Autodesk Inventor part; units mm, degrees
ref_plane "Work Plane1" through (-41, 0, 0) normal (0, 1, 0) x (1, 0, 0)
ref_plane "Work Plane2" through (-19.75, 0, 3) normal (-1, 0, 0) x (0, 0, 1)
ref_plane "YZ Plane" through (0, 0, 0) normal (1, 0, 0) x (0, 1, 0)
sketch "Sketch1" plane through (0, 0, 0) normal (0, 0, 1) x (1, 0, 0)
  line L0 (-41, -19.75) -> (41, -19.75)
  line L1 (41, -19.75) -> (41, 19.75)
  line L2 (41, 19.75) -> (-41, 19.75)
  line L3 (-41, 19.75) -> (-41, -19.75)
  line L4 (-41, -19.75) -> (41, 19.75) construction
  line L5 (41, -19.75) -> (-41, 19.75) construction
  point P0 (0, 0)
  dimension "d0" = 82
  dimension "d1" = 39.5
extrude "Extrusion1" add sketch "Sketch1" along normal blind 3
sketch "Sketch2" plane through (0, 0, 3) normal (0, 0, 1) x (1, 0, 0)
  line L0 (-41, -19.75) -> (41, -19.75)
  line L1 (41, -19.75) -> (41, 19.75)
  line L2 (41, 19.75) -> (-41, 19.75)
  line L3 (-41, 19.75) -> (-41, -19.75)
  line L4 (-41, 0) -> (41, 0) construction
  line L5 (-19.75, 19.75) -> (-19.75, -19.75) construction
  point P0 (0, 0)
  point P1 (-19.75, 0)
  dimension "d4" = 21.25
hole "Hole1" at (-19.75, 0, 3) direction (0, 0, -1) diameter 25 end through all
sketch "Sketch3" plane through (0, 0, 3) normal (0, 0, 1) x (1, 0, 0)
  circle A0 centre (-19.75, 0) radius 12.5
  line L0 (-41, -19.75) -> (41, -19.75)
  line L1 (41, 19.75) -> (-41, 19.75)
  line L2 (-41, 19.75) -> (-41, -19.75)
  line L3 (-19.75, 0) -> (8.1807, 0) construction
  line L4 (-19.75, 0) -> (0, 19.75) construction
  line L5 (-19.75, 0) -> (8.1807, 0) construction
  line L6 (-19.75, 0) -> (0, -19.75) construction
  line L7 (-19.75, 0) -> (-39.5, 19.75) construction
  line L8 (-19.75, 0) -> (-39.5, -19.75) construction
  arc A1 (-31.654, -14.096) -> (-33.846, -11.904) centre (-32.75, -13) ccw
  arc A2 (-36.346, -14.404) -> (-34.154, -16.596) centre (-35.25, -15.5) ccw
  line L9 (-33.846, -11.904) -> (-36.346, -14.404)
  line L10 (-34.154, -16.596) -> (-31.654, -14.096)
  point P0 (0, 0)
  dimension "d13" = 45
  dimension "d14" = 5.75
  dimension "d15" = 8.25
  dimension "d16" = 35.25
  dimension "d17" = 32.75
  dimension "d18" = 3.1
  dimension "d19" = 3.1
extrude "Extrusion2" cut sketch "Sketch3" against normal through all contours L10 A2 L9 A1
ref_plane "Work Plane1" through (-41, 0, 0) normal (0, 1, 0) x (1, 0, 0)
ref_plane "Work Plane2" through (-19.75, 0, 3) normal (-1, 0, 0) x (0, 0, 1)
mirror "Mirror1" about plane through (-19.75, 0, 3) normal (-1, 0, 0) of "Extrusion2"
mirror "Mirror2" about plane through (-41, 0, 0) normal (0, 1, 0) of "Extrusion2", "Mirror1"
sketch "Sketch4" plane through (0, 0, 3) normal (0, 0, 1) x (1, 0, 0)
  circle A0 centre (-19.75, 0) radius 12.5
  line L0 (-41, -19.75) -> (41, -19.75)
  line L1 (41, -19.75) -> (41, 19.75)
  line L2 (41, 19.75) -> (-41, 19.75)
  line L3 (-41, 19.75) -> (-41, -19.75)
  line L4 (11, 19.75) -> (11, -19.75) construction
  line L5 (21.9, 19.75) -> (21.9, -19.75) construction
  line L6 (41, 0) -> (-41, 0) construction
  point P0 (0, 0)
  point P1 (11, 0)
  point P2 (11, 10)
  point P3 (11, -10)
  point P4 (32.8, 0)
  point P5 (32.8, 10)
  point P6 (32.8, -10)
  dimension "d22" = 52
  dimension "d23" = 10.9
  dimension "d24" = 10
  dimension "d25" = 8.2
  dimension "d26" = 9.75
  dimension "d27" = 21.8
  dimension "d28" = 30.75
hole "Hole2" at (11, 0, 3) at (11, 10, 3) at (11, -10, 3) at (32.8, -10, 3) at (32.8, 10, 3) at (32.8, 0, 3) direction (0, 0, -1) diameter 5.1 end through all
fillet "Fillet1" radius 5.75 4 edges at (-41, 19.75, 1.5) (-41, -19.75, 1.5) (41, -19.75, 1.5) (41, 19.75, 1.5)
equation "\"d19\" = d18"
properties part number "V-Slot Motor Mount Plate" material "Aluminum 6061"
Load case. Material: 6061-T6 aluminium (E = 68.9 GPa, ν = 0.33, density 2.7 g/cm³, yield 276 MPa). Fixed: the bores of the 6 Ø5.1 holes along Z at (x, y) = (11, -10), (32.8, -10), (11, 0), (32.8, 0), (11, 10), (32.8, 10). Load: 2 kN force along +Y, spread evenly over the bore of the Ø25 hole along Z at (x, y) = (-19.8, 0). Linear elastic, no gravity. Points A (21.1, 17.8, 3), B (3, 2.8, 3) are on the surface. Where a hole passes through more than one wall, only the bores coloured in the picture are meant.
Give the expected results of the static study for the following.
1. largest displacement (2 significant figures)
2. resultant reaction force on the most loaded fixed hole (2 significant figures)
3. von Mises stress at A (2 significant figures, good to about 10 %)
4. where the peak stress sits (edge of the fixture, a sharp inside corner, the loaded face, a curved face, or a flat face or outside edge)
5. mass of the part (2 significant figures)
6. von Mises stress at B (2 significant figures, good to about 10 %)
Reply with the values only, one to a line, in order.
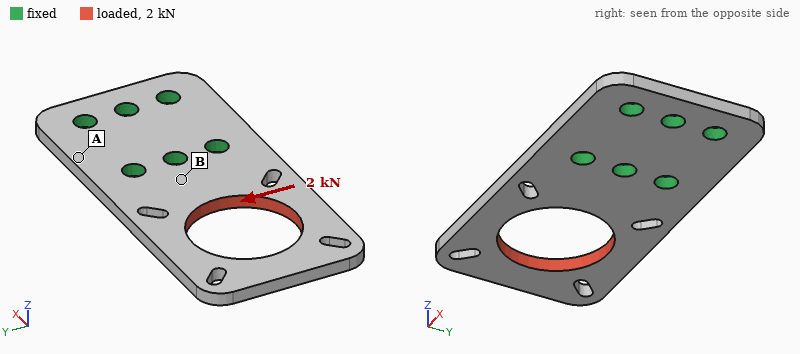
0.17 mm
2.0 kN
21 MPa
a curved face
20 g
67 MPa
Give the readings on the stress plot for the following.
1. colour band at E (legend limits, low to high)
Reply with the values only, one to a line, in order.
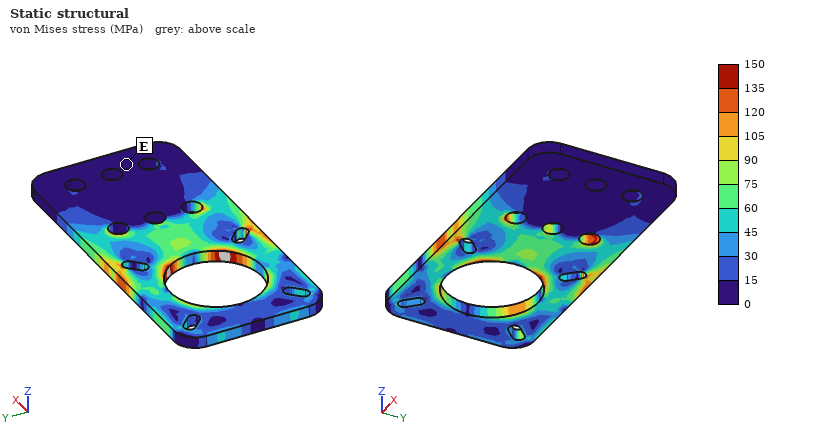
0 to 15 MPa
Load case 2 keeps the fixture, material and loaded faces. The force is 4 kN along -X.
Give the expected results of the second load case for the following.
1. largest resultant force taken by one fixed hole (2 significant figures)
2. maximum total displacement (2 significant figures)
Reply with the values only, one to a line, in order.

1.5 kN
64 µm
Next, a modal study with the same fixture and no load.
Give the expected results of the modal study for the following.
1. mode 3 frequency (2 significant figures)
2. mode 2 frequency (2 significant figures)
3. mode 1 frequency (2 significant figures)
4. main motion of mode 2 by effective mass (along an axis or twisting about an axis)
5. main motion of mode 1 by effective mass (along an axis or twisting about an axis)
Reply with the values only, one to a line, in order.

5500 Hz
2300 Hz
950 Hz
twisting about X
along Z
